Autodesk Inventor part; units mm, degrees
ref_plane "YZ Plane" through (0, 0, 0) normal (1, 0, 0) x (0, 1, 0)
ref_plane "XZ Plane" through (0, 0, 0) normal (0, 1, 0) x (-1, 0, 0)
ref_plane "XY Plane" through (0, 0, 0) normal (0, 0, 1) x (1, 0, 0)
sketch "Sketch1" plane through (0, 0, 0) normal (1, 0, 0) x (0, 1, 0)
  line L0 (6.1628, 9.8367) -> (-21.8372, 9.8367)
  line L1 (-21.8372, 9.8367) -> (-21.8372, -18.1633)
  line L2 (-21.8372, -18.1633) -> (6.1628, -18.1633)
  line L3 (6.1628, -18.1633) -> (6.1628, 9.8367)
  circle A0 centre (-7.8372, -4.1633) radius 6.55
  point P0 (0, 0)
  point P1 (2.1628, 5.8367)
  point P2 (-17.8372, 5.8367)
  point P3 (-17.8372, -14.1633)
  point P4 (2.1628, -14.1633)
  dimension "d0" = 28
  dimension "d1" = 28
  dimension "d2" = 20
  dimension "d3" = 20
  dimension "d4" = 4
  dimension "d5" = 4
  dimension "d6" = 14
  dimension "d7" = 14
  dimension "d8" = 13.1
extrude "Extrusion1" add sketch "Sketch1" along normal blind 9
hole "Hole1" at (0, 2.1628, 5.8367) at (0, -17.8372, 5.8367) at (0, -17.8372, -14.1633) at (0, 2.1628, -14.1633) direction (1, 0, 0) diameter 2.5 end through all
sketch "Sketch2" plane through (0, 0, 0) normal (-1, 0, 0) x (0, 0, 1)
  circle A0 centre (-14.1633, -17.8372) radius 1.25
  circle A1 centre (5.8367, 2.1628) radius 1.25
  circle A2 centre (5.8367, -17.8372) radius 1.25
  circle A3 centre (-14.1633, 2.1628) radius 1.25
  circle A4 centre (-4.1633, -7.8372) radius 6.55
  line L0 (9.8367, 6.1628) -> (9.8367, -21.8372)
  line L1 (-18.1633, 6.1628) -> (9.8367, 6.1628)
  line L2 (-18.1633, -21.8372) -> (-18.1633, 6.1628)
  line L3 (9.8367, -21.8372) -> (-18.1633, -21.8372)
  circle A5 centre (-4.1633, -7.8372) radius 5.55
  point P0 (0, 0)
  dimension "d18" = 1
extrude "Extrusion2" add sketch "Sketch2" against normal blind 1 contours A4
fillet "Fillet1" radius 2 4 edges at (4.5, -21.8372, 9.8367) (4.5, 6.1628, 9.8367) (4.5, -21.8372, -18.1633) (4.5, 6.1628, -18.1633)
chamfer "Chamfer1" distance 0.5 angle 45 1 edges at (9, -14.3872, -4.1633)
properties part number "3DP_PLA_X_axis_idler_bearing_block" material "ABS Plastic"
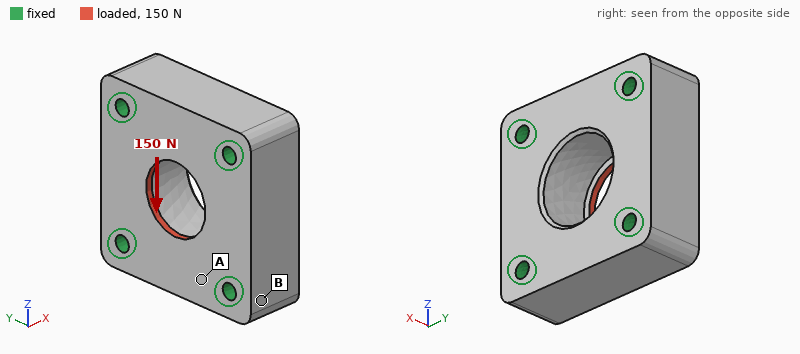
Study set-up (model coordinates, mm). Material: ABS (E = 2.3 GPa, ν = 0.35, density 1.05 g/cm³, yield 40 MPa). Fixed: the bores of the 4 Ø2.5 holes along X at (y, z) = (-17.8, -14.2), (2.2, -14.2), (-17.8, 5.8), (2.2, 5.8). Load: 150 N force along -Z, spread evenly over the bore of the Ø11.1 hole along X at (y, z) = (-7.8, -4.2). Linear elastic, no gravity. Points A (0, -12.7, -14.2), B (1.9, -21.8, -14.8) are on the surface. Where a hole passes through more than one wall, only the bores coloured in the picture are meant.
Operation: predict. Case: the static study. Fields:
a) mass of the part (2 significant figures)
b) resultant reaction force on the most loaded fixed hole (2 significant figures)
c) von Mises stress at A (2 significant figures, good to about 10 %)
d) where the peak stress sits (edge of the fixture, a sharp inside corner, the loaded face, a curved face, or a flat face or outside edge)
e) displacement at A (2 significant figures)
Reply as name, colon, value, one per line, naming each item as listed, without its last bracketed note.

mass of the part: 6.0 g
resultant reaction force on the most loaded fixed hole: 41 N
von Mises stress at A: 1.3 MPa
where the peak stress sits: a sharp inside corner
displacement at A: 4.4 µm
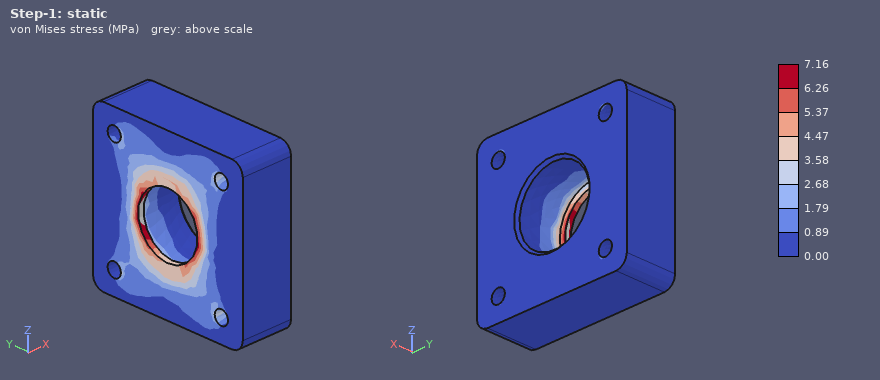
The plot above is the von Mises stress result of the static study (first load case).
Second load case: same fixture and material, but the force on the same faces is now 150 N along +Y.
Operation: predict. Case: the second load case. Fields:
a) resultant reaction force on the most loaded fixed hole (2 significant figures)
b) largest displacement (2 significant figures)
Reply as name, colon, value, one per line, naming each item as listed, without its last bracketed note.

resultant reaction force on the most loaded fixed hole: 41 N
largest displacement: 15 µm
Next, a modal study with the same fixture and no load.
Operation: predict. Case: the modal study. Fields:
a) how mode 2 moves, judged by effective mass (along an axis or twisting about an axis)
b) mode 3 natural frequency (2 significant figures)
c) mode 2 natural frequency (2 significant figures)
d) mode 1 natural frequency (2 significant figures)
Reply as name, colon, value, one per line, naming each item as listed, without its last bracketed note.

how mode 2 moves, judged by effective mass: along X
mode 3 natural frequency: 19 kHz
mode 2 natural frequency: 17 kHz
mode 1 natural frequency: 14 kHz
